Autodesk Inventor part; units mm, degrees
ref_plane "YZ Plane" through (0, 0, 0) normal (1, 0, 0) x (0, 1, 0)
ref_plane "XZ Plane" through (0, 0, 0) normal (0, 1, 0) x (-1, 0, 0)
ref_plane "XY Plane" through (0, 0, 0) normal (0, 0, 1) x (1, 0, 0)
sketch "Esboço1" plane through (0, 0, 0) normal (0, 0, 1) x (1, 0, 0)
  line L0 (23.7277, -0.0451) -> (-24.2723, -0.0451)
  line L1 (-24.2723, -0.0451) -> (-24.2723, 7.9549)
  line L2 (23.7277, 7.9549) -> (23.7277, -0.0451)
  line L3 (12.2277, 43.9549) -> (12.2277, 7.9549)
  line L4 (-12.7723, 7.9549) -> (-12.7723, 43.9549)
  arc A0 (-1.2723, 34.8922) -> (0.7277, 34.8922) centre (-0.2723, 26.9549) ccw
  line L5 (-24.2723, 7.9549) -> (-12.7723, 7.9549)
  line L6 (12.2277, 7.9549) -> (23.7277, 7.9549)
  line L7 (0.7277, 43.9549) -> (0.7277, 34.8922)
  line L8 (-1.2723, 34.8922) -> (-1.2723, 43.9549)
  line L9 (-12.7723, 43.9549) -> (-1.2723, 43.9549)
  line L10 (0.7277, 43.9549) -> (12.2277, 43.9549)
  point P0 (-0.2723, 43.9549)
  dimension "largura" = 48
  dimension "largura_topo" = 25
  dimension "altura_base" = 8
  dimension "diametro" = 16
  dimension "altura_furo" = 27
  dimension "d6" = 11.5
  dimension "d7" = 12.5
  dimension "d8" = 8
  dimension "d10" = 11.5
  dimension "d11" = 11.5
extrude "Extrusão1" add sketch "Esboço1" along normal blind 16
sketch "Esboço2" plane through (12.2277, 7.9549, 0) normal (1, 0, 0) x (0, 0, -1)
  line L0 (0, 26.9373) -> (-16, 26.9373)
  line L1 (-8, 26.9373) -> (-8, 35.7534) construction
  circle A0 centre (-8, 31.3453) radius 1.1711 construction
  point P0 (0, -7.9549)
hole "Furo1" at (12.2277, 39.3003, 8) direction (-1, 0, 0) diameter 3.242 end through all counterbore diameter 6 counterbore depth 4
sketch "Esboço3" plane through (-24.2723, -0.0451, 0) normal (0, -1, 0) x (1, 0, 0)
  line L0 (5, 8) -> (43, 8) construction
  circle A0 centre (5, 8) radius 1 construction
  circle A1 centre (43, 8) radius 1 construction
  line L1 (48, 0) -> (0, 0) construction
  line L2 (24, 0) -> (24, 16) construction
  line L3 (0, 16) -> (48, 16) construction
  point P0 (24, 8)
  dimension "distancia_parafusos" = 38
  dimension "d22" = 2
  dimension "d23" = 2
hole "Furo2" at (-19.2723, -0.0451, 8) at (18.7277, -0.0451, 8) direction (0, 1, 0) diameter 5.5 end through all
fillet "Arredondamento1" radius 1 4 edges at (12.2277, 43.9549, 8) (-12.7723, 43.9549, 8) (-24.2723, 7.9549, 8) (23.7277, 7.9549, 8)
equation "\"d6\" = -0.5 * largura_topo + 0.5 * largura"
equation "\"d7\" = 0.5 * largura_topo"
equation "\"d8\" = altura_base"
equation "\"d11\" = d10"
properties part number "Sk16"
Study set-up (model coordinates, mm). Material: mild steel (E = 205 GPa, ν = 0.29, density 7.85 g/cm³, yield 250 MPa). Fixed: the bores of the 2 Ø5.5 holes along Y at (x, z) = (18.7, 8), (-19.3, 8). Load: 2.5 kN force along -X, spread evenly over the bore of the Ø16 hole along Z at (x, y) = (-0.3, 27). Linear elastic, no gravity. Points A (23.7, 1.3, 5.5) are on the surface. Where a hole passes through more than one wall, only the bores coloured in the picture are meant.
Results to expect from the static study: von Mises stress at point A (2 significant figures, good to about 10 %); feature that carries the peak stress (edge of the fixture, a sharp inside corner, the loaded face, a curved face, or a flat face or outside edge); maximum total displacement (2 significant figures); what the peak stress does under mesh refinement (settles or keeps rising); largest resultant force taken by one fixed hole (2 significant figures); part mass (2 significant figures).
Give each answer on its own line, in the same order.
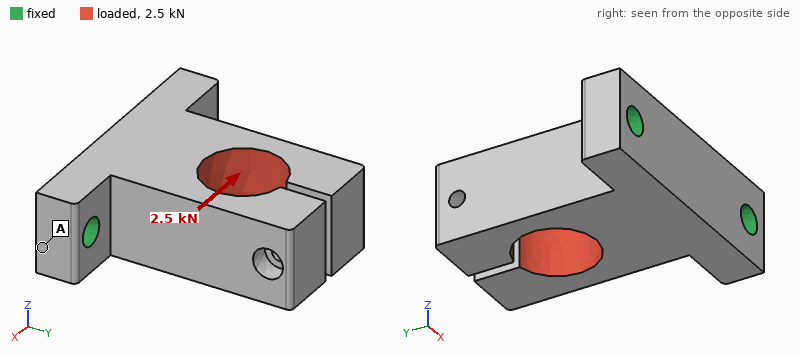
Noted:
10 MPa
edge of the fixture
44 µm
keeps rising
2.2 kN
130 g
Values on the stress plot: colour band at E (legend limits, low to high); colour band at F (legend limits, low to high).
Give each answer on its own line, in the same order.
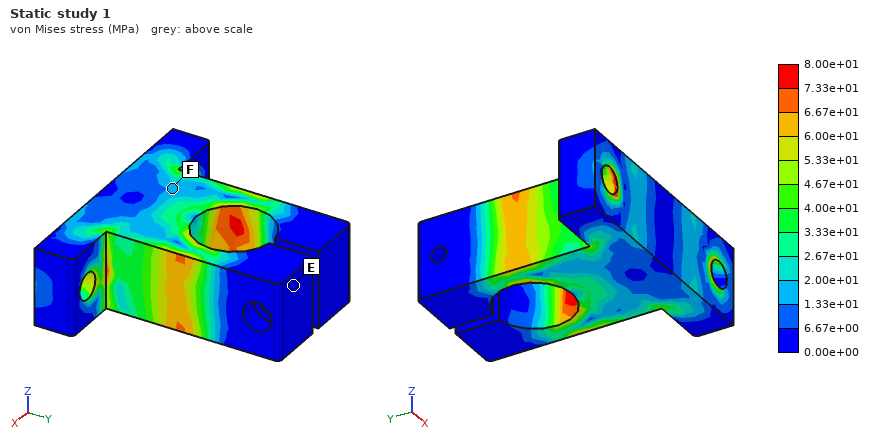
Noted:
0.00e+00 to 6.67e+00 MPa
1.33e+01 to 2.00e+01 MPa
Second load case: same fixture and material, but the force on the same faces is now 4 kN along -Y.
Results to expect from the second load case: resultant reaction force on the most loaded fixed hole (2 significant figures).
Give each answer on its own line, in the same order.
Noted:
2.1 kN
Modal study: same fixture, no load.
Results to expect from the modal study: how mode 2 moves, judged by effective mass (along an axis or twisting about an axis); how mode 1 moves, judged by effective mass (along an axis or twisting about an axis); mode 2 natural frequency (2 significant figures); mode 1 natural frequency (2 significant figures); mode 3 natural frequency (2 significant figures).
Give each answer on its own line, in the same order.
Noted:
along X
along Z
4300 Hz
4000 Hz
4500 Hz
